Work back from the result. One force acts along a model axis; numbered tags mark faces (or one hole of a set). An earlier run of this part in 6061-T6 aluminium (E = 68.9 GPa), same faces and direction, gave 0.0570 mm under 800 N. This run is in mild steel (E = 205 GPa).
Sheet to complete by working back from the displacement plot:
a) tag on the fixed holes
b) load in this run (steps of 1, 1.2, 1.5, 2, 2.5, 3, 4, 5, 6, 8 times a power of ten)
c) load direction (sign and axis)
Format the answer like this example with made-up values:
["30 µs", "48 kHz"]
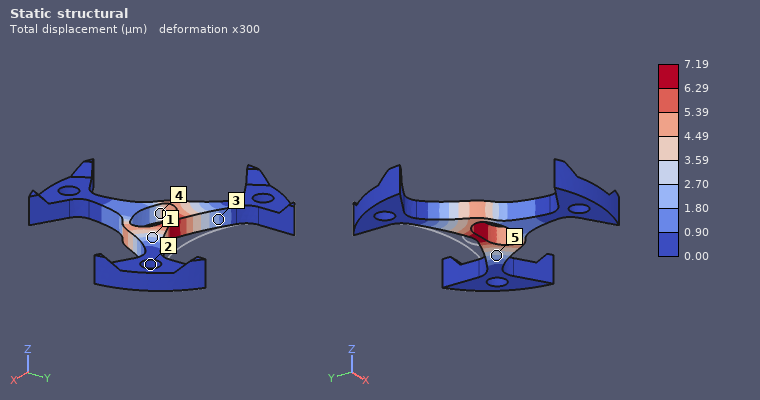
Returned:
["2", "300 N", "-Y"]
